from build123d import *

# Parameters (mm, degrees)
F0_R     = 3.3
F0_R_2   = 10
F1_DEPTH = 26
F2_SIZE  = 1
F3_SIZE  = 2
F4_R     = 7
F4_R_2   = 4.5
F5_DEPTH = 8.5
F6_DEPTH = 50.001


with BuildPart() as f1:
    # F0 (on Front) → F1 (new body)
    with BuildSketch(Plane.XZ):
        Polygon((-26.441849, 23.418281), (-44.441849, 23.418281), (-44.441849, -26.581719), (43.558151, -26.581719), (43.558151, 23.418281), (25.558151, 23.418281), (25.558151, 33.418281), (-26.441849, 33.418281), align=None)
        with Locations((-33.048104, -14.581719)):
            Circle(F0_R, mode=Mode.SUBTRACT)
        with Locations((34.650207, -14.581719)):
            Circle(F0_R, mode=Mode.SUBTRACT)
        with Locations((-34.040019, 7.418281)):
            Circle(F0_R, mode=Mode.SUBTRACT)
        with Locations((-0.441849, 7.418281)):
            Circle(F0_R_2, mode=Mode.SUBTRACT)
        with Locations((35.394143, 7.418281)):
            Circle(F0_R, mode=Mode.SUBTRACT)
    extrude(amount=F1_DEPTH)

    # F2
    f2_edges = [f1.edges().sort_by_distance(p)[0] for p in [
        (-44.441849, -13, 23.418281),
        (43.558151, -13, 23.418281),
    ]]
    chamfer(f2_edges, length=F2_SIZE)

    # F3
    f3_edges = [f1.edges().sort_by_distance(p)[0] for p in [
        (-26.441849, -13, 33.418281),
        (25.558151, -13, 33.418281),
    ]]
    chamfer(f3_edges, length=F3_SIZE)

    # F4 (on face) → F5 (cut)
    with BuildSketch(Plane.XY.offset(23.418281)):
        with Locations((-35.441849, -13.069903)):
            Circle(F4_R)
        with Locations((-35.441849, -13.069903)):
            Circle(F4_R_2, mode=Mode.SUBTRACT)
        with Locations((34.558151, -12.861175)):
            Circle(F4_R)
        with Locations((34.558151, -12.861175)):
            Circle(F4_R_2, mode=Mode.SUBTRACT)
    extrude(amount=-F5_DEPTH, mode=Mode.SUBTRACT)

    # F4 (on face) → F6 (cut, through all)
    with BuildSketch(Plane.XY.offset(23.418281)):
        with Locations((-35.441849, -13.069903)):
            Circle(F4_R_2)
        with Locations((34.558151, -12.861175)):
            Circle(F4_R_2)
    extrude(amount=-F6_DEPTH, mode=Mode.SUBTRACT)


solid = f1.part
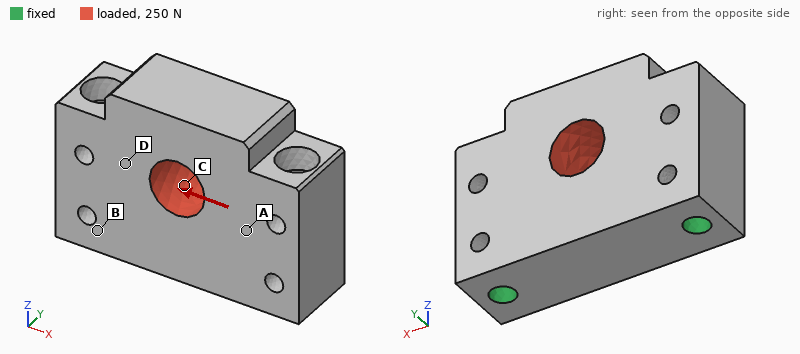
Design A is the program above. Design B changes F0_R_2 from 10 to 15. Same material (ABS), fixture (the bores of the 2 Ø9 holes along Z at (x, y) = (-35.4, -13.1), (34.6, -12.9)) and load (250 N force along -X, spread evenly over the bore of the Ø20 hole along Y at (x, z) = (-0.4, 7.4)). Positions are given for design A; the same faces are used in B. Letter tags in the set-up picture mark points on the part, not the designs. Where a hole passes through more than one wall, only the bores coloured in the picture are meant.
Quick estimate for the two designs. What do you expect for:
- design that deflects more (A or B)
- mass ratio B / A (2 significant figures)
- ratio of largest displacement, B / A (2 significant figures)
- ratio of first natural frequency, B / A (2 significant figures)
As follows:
B
0.91
1.3
1.0
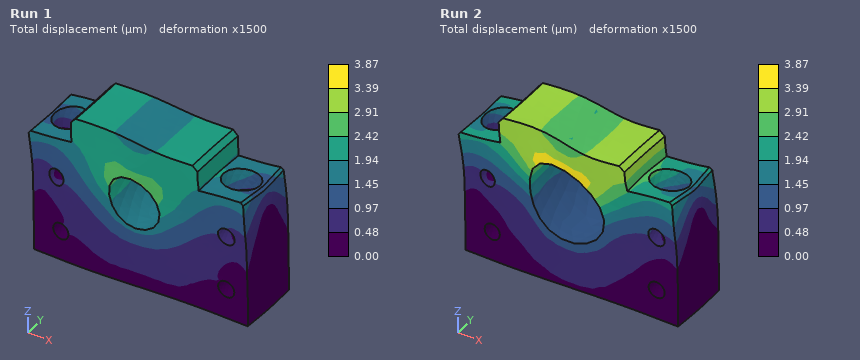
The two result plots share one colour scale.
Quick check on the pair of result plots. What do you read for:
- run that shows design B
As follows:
Run 2
